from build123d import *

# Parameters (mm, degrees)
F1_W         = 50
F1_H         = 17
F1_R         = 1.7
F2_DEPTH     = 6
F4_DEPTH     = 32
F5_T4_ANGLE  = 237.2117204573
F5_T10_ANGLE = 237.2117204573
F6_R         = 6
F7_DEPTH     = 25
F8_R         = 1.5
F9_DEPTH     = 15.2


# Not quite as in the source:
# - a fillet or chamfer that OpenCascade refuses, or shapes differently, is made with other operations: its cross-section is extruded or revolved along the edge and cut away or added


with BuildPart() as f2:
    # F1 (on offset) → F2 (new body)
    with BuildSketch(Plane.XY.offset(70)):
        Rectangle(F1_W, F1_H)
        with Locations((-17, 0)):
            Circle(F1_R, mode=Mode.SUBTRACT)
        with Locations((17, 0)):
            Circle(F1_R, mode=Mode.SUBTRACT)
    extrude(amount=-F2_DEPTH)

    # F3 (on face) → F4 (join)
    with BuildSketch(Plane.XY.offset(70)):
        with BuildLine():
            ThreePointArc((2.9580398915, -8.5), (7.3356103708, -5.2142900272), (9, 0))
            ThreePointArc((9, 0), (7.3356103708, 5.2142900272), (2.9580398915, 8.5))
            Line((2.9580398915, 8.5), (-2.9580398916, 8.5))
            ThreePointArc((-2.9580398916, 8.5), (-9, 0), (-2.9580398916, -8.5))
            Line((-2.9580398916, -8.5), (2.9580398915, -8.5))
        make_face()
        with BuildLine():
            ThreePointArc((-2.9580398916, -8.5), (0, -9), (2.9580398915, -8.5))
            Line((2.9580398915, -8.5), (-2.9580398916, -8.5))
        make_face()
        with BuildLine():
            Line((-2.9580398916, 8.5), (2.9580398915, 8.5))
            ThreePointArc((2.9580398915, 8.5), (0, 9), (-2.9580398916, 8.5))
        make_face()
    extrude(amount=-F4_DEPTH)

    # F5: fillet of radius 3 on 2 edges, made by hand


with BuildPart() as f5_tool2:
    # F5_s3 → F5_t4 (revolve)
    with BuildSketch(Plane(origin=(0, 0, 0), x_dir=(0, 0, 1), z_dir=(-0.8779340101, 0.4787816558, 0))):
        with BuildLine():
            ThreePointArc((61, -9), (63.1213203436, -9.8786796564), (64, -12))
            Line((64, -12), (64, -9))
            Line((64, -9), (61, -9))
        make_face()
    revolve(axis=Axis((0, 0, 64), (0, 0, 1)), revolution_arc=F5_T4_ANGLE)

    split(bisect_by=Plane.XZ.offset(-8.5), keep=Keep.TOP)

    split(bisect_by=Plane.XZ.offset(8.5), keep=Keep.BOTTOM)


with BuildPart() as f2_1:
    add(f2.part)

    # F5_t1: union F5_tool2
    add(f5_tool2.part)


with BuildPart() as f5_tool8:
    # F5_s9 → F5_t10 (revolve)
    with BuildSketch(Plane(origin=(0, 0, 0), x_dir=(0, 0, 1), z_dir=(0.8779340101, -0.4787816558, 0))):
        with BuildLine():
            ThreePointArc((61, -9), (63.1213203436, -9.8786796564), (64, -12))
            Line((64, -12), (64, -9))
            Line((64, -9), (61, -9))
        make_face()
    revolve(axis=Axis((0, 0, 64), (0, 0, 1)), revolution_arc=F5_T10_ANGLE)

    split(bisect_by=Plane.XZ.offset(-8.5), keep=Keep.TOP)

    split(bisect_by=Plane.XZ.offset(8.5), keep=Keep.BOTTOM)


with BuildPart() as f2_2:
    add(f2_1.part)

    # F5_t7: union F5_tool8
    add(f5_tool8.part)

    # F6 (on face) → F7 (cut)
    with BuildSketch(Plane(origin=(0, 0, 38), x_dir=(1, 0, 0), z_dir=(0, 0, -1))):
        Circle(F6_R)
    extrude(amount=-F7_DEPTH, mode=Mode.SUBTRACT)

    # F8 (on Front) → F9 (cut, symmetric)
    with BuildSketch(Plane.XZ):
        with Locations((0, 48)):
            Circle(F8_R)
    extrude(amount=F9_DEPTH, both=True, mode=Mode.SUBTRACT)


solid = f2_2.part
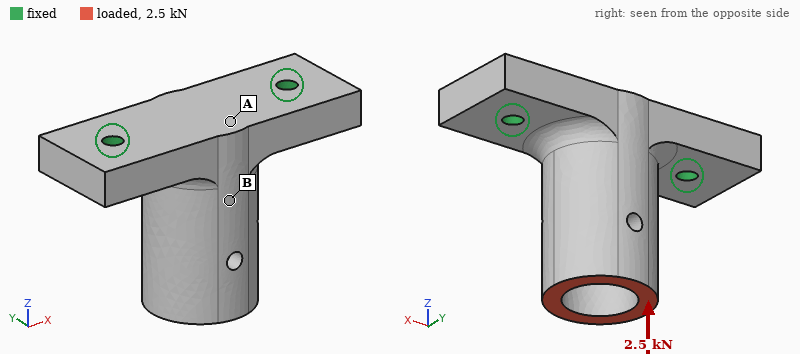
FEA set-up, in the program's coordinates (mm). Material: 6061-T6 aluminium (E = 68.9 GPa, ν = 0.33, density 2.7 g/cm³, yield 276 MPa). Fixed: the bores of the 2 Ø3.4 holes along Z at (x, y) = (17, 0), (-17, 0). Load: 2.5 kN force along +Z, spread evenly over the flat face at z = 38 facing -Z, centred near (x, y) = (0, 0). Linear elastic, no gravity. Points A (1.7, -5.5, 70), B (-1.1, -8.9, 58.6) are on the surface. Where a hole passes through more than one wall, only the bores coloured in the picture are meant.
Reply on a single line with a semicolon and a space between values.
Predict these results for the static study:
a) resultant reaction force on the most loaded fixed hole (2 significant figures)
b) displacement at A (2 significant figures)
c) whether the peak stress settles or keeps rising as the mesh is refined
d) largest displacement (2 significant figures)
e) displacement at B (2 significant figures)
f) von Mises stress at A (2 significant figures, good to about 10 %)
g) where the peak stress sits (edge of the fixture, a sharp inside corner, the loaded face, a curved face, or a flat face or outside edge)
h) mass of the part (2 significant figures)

1.3 kN; 16 µm; keeps rising; 21 µm; 17 µm; 25 MPa; edge of the fixture; 24 g
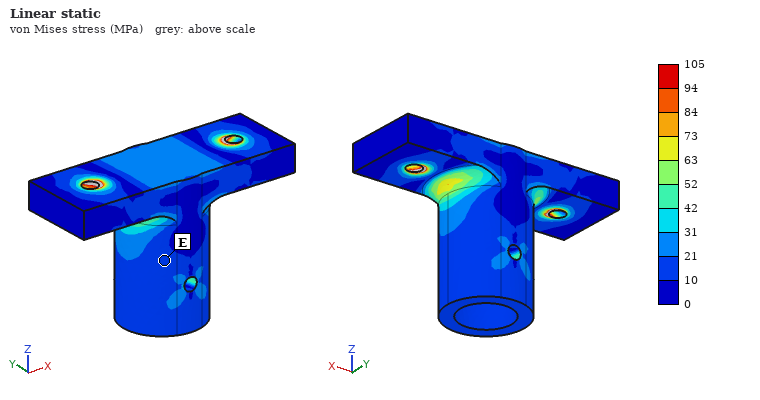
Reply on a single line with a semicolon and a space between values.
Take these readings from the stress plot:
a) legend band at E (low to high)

10 to 21 MPa
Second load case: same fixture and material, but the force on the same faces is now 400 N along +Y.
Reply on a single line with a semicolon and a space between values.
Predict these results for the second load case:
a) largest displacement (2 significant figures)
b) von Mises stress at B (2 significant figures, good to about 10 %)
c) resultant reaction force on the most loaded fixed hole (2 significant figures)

83 µm; 14 MPa; 200 N
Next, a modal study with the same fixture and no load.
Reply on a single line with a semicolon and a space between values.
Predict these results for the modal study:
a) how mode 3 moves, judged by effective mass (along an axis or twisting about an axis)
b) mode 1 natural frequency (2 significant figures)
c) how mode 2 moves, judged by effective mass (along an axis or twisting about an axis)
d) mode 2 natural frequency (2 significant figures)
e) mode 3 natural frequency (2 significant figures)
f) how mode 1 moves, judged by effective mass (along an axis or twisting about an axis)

along Z; 5700 Hz; along X; 12 kHz; 16 kHz; along Y
